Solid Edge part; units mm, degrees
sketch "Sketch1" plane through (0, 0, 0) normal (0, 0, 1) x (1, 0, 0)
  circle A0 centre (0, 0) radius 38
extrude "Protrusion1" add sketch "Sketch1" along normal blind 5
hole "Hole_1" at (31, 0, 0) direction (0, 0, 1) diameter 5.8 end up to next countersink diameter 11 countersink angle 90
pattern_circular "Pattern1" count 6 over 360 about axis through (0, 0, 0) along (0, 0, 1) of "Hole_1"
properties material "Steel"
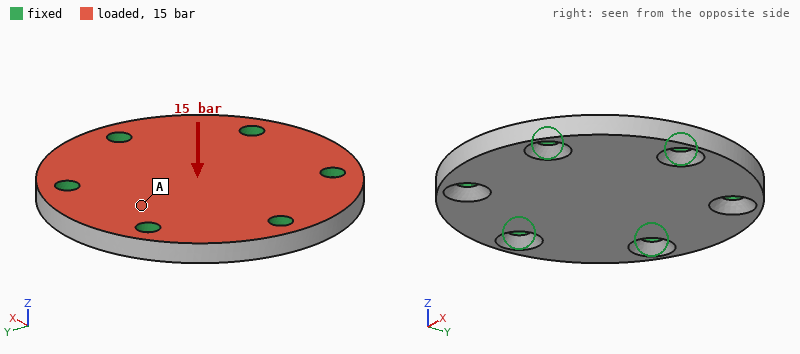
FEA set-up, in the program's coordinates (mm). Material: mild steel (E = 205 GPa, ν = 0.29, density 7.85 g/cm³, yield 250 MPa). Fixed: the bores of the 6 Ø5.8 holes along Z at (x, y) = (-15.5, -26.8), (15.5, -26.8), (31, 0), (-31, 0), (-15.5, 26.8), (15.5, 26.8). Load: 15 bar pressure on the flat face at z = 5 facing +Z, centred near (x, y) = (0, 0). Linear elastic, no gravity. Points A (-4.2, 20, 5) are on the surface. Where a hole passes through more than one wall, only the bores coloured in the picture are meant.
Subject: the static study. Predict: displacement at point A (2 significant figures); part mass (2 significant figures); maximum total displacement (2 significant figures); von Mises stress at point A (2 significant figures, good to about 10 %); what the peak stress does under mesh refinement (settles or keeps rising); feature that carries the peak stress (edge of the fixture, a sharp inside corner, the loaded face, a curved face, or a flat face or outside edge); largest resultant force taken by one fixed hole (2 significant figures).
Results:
6.7 µm
170 g
14 µm
18 MPa
keeps rising
edge of the fixture
1.2 kN
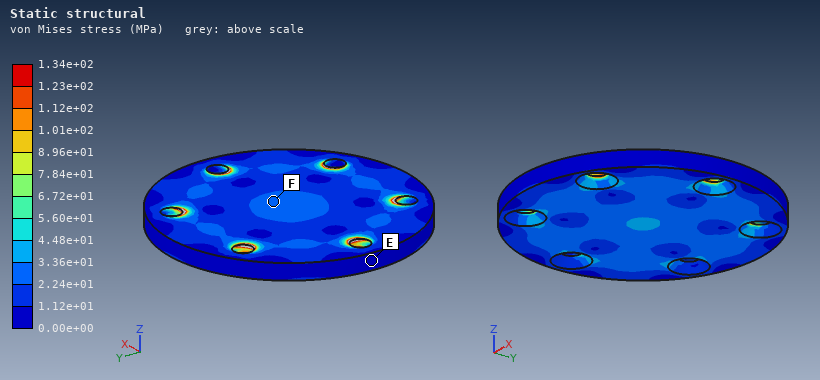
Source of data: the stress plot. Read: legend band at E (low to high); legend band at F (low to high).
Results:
0.00e+00 to 1.12e+01 MPa
2.24e+01 to 3.36e+01 MPa
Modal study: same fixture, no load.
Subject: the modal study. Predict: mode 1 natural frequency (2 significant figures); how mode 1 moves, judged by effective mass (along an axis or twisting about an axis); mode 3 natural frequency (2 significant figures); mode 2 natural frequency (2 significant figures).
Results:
9800 Hz
along Z
18 kHz
18 kHz
